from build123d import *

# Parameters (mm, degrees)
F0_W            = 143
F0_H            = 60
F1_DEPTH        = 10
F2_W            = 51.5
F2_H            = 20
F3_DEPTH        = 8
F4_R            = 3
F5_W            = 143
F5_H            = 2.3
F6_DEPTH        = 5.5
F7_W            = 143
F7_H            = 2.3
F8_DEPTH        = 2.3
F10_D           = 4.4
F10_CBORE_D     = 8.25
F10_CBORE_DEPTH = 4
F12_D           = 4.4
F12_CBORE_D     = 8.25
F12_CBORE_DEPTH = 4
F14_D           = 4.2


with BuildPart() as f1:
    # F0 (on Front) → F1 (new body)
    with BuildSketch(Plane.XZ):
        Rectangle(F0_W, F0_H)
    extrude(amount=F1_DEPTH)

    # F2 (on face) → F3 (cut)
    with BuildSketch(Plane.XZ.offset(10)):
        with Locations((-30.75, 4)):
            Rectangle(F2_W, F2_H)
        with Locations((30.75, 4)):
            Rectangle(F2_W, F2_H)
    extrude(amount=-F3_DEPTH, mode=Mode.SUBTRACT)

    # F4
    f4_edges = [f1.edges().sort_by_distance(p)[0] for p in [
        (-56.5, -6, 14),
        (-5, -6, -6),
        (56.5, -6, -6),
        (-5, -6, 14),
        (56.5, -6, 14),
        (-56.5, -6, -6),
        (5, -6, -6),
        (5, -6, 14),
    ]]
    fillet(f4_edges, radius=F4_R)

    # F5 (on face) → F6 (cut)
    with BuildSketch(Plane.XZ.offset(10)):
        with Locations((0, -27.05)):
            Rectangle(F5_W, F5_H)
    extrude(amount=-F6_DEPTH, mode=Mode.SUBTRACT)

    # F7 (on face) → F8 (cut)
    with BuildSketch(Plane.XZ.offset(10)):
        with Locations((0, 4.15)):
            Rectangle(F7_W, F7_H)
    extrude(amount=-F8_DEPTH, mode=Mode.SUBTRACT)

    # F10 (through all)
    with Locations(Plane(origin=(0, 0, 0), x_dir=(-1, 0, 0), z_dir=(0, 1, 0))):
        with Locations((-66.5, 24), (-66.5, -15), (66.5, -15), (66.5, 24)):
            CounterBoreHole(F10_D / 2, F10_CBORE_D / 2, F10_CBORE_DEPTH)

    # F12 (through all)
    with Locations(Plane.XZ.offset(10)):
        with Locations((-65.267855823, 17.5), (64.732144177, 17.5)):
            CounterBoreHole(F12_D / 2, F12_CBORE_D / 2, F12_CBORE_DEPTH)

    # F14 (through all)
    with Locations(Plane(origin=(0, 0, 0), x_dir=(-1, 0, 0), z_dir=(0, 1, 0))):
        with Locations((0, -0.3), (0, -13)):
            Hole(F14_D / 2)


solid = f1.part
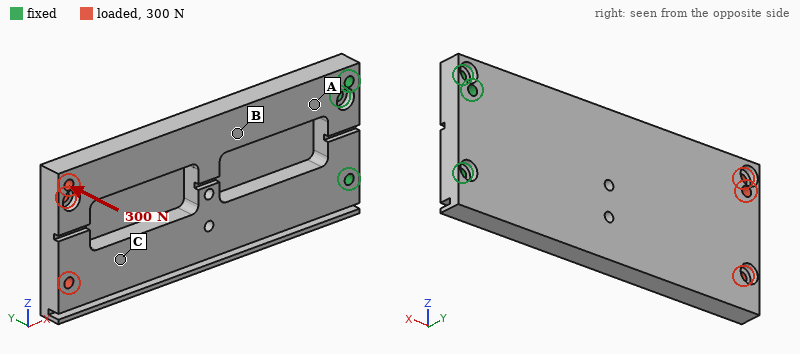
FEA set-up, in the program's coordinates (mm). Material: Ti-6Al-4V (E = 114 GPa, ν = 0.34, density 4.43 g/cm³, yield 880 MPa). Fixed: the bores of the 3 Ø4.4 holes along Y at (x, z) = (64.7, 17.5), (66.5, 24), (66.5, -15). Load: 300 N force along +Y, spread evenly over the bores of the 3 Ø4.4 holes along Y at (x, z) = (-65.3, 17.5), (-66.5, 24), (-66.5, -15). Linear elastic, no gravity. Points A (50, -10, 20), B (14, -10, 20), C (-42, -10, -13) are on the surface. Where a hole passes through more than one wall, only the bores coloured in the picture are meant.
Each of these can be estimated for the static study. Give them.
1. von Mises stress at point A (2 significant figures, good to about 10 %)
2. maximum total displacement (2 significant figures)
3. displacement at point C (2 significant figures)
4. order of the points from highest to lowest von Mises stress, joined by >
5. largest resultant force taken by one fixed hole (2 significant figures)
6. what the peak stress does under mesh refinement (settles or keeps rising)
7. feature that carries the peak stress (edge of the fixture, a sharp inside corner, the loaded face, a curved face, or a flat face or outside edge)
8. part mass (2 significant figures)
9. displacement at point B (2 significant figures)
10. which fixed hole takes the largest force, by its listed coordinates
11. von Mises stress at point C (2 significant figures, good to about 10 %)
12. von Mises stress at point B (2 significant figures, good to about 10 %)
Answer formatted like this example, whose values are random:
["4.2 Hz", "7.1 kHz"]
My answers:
["55 MPa", "0.68 mm", "0.46 mm", "A > B > C", "2.3 kN", "keeps rising", "edge of the fixture", "290 g", "0.15 mm", "(64.7, 17.5)", "12 MPa", "35 MPa"]
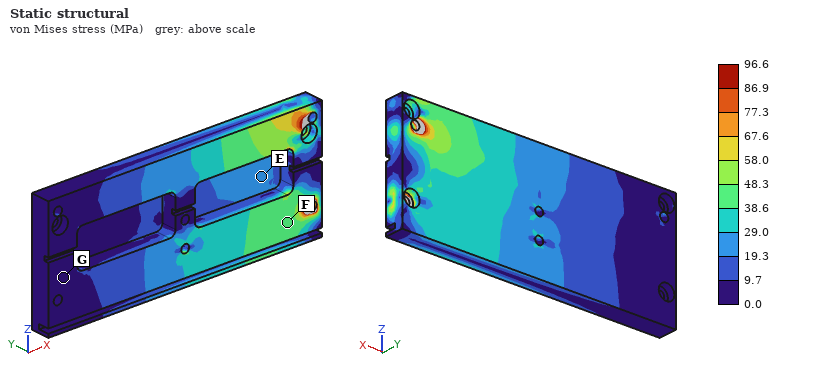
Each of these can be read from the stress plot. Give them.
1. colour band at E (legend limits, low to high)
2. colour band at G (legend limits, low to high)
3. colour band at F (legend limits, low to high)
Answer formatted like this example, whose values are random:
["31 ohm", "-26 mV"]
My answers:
["19.3 to 29.0 MPa", "0.0 to 9.7 MPa", "38.6 to 48.3 MPa"]
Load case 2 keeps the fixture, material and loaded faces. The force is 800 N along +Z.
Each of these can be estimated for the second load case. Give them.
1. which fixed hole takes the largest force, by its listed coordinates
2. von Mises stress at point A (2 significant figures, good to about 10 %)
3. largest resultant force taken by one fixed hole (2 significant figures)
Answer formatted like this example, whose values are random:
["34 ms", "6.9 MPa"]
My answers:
["(66.5, -15)", "17 MPa", "2.6 kN"]
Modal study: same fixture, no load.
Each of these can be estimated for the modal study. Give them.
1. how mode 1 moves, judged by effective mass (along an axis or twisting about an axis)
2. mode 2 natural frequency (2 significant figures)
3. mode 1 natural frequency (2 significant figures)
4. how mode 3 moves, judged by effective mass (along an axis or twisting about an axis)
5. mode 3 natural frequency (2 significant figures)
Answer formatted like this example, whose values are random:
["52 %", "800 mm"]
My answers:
["along Y", "1400 Hz", "390 Hz", "along Z", "2000 Hz"]
